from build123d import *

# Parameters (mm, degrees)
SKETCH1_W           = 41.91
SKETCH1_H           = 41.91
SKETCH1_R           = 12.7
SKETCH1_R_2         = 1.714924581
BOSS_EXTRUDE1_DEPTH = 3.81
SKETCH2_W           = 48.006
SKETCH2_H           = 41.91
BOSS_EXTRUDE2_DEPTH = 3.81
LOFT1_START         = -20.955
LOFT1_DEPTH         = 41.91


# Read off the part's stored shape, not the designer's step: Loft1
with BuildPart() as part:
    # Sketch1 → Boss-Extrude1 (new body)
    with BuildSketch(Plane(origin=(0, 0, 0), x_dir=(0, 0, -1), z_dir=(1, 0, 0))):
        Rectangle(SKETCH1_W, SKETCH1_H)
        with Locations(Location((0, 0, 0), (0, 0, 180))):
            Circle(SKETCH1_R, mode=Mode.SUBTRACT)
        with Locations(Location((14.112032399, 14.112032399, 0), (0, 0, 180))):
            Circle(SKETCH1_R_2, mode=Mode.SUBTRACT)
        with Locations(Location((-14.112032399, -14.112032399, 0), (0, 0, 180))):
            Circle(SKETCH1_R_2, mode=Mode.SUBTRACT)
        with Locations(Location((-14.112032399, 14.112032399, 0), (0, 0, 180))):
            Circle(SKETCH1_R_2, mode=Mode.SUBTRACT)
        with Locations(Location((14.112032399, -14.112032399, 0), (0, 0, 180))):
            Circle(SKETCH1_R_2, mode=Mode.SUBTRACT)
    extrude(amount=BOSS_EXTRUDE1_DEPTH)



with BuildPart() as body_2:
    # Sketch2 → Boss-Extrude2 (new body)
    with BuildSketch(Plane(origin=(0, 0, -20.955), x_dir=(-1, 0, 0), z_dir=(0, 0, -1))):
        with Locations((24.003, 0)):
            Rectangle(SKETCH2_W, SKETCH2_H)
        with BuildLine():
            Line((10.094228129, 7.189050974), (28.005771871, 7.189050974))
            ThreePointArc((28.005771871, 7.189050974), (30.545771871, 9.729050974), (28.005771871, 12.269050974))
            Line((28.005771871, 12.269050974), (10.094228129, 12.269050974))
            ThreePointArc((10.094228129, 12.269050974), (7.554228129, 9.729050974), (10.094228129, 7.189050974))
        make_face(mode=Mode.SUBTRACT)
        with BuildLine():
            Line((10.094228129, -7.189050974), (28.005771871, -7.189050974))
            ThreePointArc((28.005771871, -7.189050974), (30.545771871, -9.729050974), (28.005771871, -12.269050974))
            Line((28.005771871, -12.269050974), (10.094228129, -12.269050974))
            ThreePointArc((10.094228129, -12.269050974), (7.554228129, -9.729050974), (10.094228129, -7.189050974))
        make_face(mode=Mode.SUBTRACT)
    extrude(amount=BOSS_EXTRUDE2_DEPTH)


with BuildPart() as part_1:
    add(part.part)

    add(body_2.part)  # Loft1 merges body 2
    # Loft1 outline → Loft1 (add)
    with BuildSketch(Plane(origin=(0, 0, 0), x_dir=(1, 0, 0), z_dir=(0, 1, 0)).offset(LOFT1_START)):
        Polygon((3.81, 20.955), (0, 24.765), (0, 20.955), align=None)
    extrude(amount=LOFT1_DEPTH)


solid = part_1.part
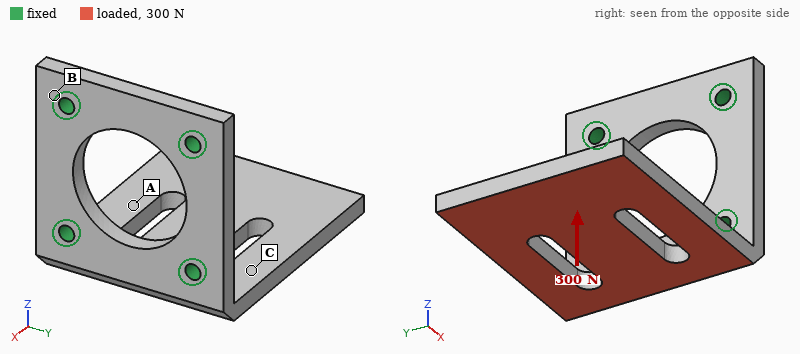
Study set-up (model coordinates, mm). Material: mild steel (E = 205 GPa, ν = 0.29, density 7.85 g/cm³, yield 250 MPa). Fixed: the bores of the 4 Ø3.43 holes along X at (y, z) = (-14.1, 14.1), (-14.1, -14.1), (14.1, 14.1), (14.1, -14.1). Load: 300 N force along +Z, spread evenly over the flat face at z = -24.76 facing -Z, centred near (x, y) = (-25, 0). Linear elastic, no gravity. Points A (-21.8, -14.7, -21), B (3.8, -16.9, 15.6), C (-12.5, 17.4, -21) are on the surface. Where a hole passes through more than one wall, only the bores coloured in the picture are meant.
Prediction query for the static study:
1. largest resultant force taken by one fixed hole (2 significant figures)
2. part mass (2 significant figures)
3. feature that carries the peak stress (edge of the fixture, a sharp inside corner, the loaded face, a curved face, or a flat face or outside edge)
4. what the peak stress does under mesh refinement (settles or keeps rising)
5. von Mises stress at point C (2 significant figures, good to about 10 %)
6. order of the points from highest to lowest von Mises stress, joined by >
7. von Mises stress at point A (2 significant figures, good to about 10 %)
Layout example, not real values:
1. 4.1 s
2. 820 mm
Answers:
1. 170 N
2. 92 g
3. edge of the fixture
4. keeps rising
5. 51 MPa
6. C > A > B
7. 30 MPa
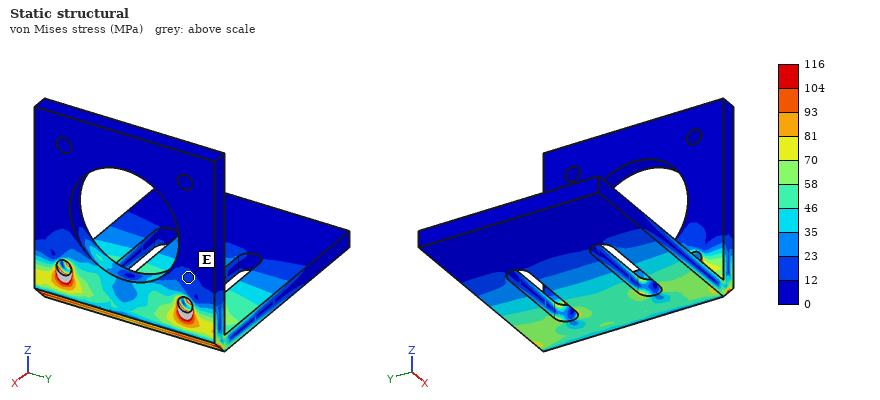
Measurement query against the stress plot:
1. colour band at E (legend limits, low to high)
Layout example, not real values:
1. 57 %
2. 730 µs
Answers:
1. 12 to 23 MPa
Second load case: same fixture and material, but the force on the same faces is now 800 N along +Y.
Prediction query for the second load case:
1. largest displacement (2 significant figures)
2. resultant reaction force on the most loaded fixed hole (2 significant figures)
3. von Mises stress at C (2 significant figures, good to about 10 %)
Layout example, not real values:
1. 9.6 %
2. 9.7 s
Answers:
1. 35 µm
2. 850 N
3. 24 MPa
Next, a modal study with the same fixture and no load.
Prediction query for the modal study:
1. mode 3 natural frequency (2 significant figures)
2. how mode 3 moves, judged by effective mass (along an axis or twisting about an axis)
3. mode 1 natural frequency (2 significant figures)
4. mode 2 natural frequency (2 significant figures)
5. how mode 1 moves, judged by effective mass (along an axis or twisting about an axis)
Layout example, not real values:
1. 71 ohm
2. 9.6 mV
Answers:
1. 4000 Hz
2. along Y
3. 910 Hz
4. 2700 Hz
5. along Z
